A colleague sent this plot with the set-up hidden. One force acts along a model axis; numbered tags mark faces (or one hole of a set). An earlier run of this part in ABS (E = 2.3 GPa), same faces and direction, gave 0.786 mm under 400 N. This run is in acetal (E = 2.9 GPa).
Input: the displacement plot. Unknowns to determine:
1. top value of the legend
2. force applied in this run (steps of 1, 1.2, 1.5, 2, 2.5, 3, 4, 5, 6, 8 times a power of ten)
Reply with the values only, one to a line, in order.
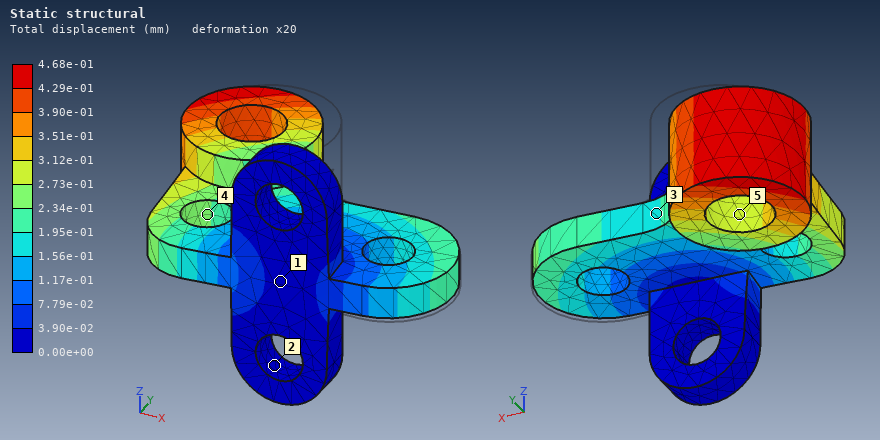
4.68e-01 mm
300 N
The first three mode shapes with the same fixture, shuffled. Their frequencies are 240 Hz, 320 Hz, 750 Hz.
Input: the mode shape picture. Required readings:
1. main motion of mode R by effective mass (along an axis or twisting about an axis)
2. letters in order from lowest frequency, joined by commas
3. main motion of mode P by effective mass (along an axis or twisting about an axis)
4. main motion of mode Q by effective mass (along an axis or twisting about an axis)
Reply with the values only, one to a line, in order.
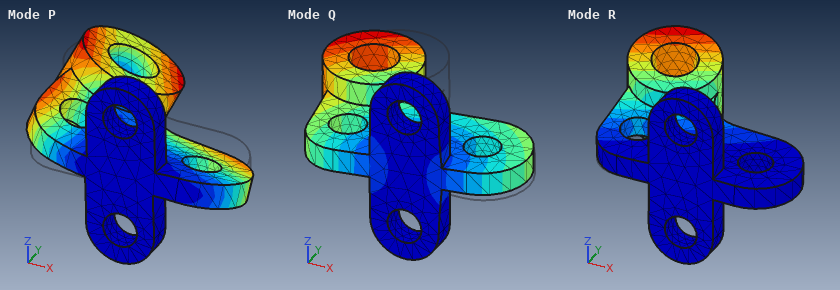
along Z
R, Q, P
twisting about Y
along X
